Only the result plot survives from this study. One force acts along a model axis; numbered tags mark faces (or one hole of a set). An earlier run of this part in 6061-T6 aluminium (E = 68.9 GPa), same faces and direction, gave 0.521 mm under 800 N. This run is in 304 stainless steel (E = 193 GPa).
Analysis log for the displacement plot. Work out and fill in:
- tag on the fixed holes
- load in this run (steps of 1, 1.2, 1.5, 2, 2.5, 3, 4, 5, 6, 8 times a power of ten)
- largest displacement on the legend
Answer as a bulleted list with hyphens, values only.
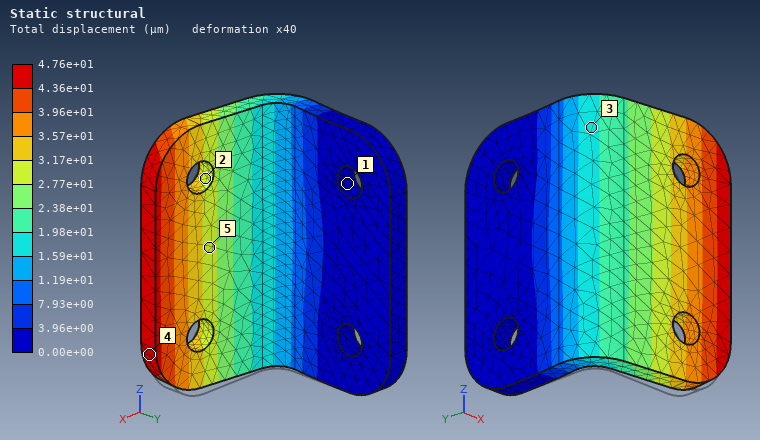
- 1
- 200 N
- 4.76e+01 µm
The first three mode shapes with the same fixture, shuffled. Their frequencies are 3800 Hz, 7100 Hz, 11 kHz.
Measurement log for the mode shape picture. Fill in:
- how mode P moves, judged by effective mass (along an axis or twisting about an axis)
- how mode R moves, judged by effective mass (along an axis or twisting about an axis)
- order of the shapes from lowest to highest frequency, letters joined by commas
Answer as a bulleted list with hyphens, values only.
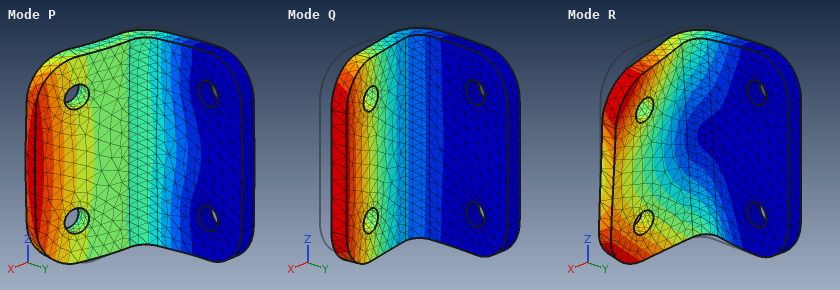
- along X
- along Z
- Q, R, P
